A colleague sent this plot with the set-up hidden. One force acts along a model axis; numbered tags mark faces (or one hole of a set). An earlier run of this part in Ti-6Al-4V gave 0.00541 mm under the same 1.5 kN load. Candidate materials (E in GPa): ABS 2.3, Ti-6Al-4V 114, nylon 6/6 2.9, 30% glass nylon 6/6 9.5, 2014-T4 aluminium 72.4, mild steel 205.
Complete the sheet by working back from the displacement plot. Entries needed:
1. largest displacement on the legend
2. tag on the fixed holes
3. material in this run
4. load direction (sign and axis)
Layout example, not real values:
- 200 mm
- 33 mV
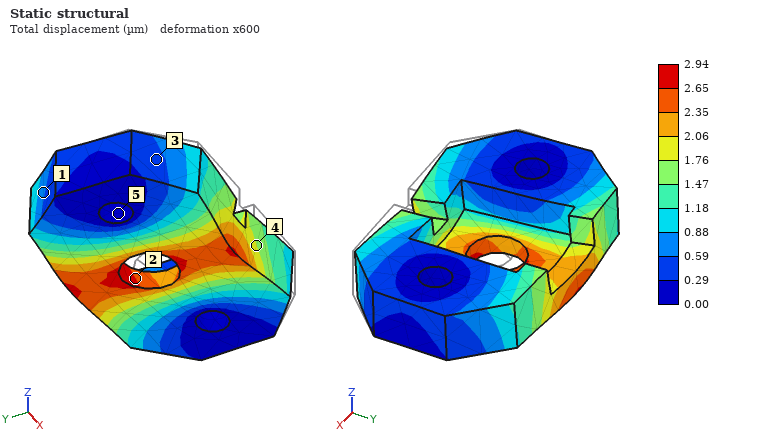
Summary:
- 2.94 µm
- 5
- mild steel
- +Y
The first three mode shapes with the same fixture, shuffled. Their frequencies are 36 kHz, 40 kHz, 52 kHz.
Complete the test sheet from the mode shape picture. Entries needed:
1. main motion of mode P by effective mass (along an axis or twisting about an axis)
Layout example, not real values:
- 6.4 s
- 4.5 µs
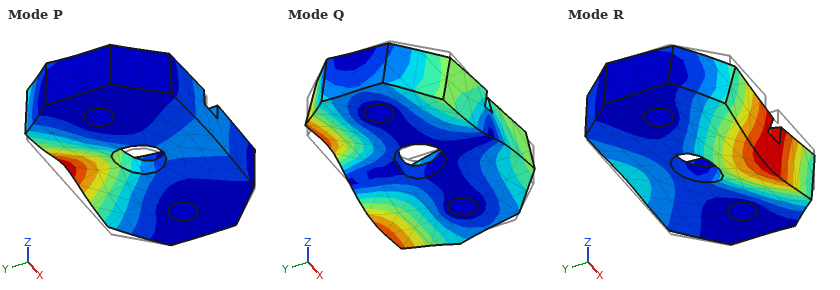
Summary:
- along Z
